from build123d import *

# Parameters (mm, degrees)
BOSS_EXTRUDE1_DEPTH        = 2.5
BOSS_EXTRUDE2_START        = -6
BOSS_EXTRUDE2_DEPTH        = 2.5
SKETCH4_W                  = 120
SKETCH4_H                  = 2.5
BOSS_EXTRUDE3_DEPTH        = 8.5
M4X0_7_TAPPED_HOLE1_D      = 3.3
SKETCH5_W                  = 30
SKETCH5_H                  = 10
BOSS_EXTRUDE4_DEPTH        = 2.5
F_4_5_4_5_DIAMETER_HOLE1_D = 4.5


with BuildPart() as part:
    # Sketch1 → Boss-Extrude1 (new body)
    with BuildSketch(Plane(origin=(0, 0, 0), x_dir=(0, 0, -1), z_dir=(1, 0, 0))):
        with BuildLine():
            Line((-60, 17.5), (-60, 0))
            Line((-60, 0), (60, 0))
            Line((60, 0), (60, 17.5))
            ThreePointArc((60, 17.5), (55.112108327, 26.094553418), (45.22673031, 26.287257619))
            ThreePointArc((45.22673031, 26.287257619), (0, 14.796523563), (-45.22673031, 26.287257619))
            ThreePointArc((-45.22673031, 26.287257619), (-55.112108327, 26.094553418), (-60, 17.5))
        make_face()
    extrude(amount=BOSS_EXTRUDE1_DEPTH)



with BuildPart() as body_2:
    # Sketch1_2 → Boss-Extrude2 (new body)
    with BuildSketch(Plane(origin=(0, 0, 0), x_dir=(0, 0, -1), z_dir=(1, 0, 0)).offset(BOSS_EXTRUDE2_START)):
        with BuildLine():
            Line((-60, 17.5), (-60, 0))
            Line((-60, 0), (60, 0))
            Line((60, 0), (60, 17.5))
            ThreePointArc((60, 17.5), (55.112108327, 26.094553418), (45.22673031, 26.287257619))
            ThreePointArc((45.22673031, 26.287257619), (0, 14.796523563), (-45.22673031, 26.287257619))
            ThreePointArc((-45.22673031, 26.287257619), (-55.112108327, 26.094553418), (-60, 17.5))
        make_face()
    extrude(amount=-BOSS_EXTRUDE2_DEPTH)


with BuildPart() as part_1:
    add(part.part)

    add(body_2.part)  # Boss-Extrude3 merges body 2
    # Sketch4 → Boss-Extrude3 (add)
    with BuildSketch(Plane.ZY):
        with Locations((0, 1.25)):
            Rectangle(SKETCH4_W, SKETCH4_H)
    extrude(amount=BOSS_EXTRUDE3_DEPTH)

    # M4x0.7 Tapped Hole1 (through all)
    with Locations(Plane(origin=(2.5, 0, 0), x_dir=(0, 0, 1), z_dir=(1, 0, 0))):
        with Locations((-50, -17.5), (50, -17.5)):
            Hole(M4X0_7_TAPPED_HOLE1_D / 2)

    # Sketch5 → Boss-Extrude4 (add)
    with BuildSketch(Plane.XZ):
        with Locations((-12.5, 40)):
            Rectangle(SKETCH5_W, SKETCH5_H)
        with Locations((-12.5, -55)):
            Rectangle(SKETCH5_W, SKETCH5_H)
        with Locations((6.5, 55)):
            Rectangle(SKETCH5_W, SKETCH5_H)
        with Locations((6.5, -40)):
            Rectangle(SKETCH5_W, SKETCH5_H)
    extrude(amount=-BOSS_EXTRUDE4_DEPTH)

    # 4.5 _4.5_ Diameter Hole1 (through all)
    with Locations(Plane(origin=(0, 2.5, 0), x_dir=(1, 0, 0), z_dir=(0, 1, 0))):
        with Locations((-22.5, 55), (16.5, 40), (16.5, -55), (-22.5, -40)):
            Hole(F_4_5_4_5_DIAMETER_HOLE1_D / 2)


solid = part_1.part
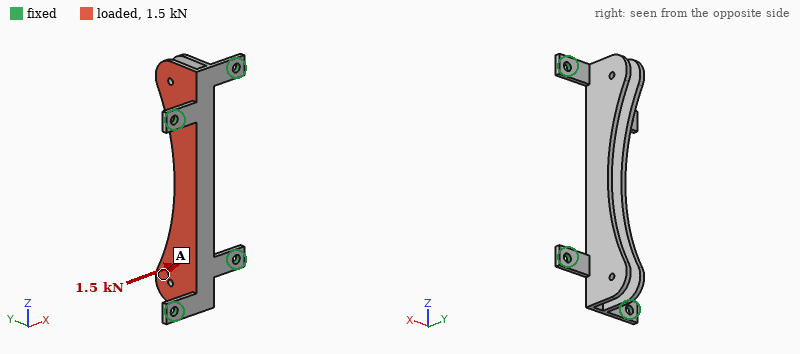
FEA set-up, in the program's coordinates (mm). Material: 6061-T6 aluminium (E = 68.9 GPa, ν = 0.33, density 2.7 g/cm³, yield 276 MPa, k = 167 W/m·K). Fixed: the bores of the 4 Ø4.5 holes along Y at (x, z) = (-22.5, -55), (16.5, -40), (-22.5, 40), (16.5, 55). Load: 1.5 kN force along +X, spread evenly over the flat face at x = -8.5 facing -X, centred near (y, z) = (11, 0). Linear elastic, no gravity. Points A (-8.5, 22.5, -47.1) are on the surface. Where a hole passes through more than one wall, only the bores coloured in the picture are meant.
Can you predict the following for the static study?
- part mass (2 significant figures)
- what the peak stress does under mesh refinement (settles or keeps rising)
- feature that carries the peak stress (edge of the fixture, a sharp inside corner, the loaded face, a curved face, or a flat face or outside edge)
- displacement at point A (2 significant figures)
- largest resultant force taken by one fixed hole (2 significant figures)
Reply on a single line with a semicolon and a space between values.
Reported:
42 g; keeps rising; edge of the fixture; 0.39 mm; 790 N
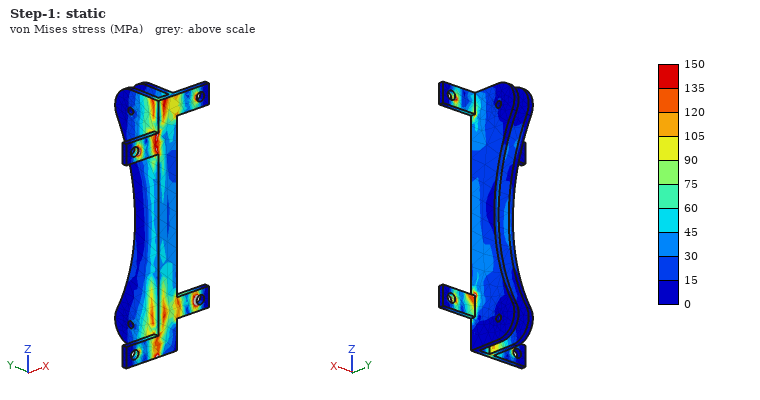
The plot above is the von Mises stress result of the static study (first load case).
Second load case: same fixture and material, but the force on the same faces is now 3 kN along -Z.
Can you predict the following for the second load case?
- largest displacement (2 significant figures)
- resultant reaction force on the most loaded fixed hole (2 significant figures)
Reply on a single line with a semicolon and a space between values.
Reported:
0.14 mm; 800 N
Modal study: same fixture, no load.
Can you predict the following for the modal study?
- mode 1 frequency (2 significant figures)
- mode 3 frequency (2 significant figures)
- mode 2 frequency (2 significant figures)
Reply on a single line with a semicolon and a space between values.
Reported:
2400 Hz; 3000 Hz; 2500 Hz
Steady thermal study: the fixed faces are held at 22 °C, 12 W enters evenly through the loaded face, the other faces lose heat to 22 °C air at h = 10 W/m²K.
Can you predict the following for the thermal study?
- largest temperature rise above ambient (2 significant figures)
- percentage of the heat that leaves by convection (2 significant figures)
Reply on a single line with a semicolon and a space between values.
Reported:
15 K; 9.7 %
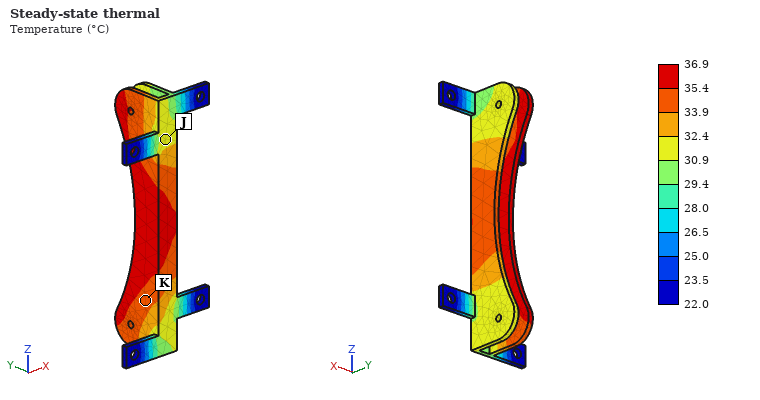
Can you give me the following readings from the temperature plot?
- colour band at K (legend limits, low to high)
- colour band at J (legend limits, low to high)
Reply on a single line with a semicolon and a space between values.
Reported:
33.9 to 35.4 °C; 30.9 to 32.4 °C
